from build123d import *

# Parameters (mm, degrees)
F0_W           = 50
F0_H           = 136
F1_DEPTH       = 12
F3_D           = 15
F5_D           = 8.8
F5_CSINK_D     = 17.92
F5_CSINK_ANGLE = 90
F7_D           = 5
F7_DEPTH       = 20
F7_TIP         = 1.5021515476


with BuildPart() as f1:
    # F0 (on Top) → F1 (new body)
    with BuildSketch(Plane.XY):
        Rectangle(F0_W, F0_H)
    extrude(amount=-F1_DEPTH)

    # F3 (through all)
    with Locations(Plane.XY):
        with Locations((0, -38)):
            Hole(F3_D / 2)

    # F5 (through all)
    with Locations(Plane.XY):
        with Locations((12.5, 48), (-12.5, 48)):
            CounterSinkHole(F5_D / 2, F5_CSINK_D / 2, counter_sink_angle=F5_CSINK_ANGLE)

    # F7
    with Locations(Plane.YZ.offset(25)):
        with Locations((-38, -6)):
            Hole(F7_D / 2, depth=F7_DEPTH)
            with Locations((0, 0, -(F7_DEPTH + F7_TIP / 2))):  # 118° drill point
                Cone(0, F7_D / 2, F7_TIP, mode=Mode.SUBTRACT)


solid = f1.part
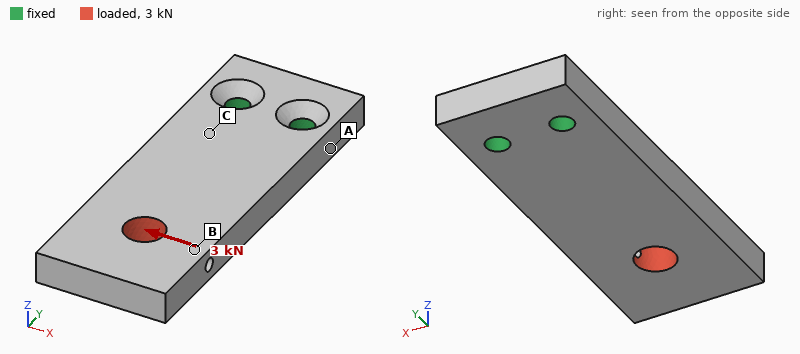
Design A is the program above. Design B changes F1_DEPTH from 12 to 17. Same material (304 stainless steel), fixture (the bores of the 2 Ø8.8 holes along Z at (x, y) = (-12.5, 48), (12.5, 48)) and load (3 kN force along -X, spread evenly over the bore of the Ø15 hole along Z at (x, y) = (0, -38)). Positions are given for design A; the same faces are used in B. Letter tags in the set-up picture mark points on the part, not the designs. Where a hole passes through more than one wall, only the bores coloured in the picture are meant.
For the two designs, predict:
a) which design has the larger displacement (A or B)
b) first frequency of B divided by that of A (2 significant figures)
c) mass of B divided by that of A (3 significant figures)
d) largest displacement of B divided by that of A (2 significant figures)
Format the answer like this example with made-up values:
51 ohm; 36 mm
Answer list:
A; 1.4; 1.42; 0.68
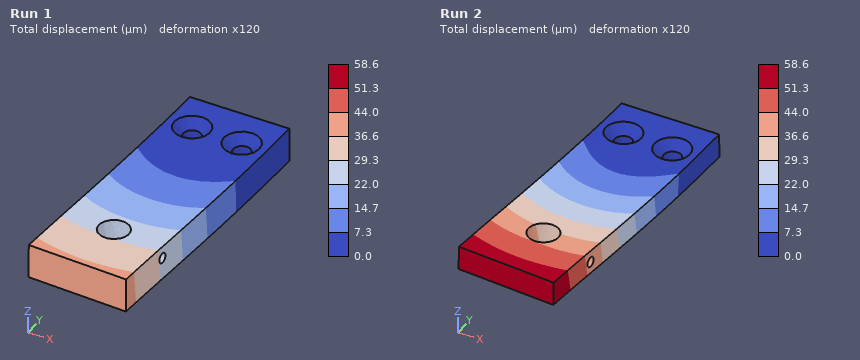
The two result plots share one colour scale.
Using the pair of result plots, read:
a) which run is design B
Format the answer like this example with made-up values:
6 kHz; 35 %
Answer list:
Run 1
